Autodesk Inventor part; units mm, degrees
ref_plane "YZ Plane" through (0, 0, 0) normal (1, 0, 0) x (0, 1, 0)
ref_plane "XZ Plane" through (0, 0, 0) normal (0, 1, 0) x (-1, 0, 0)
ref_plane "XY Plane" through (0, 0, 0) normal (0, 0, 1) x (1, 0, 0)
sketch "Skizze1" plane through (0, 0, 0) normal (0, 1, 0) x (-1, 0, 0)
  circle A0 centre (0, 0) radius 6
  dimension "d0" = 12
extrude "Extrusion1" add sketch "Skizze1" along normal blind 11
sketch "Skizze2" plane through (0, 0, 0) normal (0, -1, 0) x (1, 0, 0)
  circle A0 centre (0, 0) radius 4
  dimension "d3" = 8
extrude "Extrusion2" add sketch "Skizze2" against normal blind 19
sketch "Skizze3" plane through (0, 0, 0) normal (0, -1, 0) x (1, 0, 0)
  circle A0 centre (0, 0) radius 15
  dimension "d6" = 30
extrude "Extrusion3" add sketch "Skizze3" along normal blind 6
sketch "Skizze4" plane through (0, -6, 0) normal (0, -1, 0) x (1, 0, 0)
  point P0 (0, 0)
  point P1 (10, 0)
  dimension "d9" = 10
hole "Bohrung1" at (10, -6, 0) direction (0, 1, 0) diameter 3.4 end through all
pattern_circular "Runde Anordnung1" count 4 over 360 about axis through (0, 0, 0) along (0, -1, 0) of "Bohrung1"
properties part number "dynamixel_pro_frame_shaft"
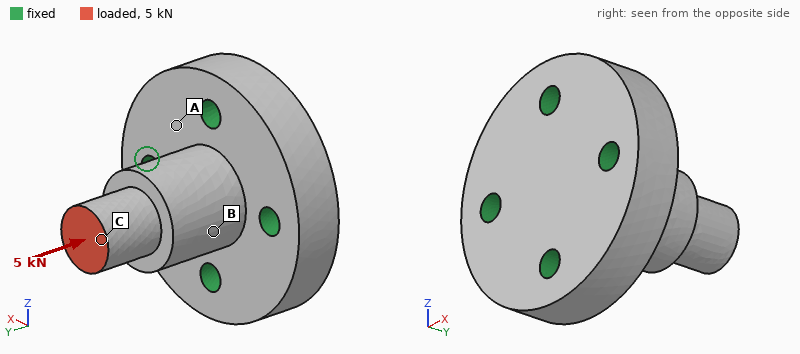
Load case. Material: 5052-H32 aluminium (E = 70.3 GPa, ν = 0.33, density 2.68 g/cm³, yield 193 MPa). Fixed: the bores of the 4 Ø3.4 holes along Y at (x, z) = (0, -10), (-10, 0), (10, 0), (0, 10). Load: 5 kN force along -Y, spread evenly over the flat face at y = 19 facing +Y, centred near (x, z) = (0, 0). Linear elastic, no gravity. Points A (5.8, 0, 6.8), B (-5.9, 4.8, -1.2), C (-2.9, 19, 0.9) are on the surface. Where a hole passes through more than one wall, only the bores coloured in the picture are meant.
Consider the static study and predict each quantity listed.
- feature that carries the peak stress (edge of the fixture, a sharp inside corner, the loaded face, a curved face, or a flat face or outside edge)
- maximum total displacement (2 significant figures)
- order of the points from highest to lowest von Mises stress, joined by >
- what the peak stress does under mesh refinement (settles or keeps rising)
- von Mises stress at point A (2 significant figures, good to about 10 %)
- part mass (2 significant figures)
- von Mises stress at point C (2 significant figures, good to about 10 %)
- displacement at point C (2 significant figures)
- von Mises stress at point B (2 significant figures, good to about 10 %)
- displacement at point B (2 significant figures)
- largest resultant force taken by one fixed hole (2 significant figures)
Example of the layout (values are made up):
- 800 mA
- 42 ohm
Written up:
- edge of the fixture
- 26 µm
- C > B > A
- keeps rising
- 16 MPa
- 15 g
- 100 MPa
- 25 µm
- 40 MPa
- 9.0 µm
- 1.3 kN
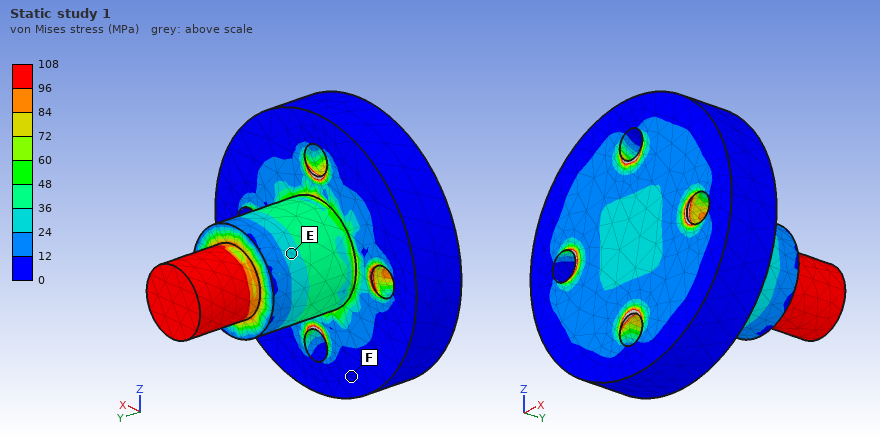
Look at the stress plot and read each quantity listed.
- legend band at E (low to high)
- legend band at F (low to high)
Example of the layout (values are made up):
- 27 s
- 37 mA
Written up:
- 24 to 36 MPa
- 0 to 12 MPa
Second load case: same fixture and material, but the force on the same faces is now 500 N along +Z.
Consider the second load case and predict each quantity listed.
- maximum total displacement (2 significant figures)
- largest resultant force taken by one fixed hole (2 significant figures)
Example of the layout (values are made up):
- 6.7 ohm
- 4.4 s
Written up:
- 40 µm
- 600 N
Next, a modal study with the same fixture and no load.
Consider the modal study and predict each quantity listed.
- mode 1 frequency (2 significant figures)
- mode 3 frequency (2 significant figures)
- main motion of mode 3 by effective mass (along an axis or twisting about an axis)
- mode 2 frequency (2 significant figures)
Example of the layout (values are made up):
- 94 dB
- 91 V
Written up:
- 20 kHz
- 49 kHz
- along Y
- 20 kHz
